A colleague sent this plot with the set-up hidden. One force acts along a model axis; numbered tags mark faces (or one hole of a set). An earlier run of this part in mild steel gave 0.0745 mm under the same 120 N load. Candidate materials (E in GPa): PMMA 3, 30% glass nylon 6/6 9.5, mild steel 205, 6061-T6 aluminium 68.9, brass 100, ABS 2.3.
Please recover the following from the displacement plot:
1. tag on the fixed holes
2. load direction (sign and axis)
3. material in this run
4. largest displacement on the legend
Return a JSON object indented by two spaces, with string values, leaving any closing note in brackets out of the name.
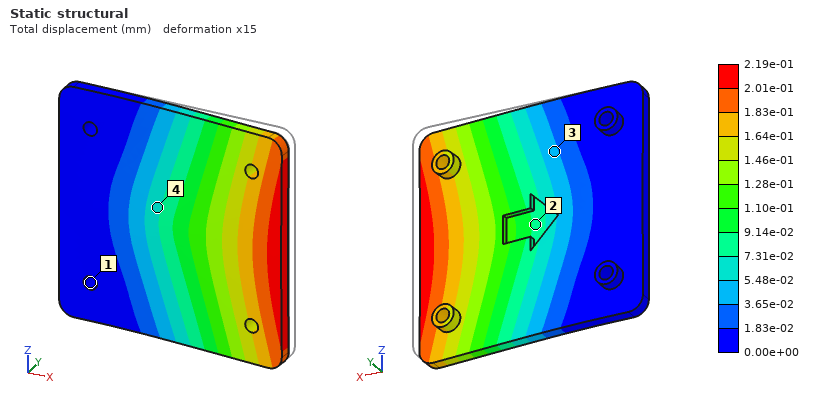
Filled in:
{
  "tag on the fixed holes": "1",
  "load direction": "-Y",
  "material in this run": "6061-T6 aluminium",
  "largest displacement on the legend": "2.19e-01 mm"
}
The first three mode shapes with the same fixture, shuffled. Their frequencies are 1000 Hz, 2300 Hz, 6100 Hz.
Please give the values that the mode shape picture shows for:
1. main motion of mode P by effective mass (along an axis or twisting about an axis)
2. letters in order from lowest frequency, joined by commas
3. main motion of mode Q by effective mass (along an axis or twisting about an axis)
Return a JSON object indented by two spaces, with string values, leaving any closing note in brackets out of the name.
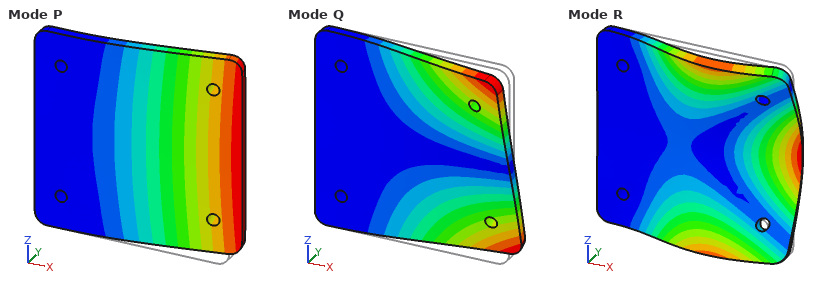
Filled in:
{
  "main motion of mode P by effective mass": "along Y",
  "letters in order from lowest frequency, joined by commas": "P, Q, R",
  "main motion of mode Q by effective mass": "twisting about X"
}
